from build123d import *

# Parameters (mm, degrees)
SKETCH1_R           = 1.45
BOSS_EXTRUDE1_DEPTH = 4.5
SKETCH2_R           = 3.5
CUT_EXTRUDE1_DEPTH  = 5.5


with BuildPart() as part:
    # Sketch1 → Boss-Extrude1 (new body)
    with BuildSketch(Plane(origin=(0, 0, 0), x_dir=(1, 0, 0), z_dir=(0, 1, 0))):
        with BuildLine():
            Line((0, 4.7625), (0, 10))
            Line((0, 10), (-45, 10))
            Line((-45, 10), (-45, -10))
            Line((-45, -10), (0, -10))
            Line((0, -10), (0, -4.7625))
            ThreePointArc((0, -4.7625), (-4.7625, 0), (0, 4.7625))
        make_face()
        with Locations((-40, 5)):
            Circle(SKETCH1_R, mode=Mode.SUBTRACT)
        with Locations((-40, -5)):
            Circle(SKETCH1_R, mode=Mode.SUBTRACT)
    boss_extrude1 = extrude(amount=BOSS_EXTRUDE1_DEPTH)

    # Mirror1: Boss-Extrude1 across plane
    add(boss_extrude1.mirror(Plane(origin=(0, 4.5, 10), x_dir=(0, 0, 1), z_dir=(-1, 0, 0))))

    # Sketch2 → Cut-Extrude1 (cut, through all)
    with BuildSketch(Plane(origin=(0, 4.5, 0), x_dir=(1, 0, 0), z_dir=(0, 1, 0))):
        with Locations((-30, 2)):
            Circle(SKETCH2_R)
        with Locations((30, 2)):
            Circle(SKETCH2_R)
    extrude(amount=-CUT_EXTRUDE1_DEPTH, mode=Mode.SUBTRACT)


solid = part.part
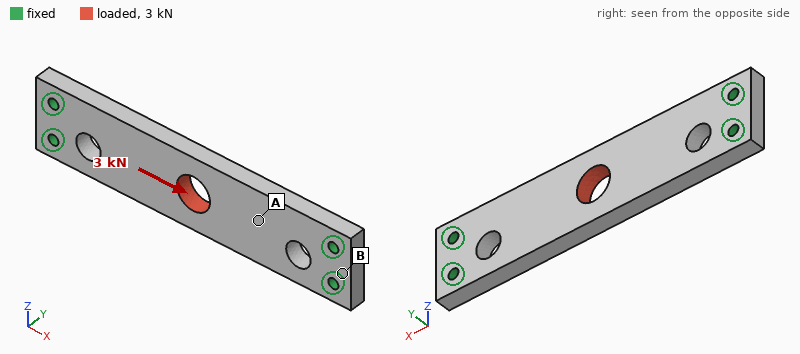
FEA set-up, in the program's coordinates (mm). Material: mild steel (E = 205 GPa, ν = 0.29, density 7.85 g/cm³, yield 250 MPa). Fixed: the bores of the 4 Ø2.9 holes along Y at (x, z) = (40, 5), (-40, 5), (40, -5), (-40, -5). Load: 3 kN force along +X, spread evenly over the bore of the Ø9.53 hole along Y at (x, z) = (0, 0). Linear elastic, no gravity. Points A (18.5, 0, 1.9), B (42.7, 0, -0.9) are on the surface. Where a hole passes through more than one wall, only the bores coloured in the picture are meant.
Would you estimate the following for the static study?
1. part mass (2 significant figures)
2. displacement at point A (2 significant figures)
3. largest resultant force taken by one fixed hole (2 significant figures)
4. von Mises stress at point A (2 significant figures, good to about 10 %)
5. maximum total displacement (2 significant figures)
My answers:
57 g
2.4 µm
840 N
16 MPa
4.1 µm
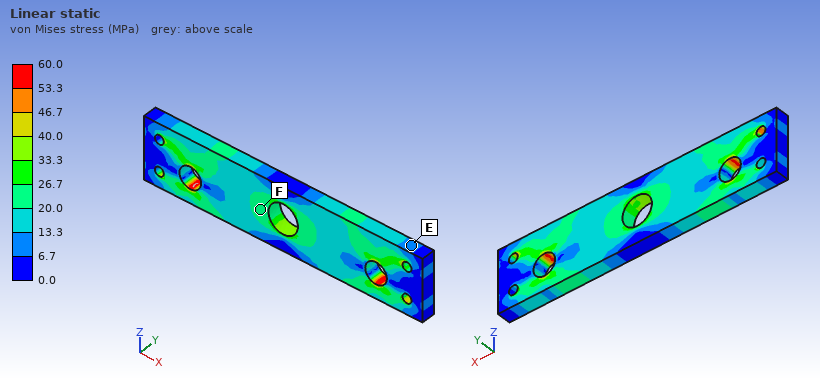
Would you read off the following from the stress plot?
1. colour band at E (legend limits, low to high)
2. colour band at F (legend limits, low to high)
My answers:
6.7 to 13.3 MPa
20.0 to 26.7 MPa
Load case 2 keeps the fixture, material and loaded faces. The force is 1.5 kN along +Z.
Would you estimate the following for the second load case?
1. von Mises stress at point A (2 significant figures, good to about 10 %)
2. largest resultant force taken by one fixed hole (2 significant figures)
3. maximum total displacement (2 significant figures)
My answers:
21 MPa
1.2 kN
14 µm
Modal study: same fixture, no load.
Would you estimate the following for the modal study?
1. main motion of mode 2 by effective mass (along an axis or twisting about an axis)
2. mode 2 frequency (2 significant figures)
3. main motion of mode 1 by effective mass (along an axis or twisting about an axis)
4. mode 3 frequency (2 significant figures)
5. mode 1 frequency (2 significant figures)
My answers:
twisting about X
8500 Hz
along Y
9700 Hz
3500 Hz
